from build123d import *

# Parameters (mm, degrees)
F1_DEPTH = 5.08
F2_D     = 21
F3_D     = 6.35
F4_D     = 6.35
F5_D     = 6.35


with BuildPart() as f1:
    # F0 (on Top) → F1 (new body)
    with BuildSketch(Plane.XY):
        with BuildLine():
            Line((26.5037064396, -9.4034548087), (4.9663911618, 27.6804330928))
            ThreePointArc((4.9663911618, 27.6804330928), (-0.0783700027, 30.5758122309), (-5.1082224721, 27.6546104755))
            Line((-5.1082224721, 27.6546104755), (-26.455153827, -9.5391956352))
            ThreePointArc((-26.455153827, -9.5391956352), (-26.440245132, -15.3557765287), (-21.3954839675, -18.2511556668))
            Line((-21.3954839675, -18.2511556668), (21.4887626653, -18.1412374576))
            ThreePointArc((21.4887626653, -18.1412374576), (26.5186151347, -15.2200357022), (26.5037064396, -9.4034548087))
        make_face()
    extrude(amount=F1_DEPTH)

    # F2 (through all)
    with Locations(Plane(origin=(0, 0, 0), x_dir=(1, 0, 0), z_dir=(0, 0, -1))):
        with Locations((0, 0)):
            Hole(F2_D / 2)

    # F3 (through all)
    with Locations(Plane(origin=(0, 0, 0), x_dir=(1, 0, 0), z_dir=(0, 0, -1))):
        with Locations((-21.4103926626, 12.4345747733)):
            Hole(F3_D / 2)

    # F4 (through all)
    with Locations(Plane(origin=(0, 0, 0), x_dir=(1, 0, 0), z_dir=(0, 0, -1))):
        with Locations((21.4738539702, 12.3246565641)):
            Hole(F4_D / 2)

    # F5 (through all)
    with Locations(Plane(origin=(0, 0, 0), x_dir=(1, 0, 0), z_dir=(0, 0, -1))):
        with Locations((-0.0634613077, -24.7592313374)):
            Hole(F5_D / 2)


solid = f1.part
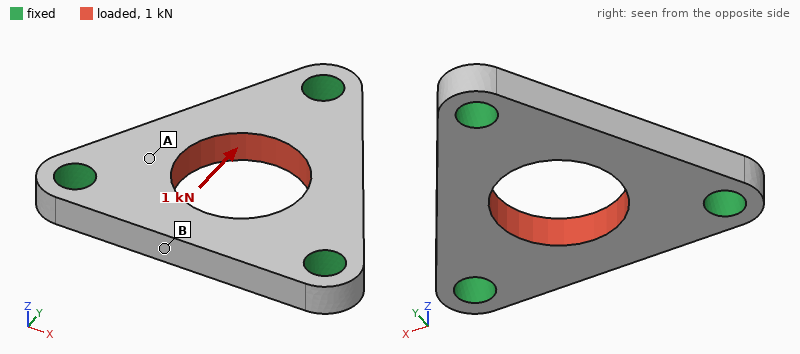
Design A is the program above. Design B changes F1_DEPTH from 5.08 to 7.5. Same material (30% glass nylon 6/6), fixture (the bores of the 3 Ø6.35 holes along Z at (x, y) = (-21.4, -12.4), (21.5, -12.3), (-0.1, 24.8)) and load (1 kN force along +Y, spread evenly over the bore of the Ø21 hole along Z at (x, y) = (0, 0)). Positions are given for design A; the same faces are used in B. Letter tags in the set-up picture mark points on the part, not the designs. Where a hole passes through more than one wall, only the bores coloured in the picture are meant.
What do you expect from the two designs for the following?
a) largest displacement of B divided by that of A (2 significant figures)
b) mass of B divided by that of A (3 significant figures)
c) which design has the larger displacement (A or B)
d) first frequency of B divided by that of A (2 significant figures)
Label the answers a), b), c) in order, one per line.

a) 0.68
b) 1.48
c) A
d) 1.3
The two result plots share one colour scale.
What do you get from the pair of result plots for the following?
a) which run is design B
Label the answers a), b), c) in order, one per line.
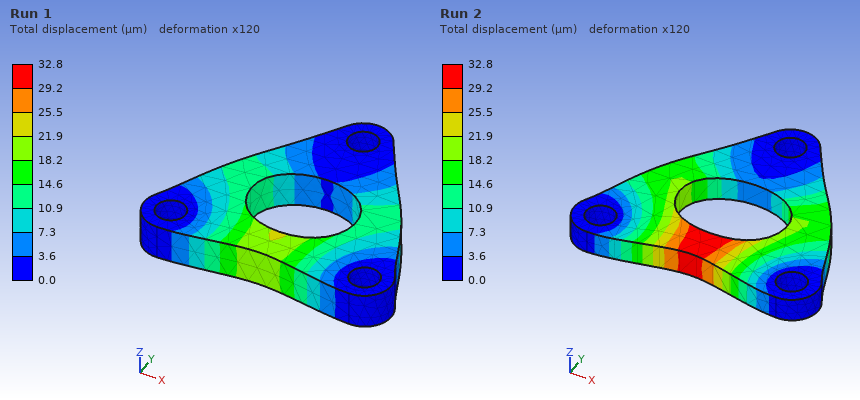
a) Run 1
